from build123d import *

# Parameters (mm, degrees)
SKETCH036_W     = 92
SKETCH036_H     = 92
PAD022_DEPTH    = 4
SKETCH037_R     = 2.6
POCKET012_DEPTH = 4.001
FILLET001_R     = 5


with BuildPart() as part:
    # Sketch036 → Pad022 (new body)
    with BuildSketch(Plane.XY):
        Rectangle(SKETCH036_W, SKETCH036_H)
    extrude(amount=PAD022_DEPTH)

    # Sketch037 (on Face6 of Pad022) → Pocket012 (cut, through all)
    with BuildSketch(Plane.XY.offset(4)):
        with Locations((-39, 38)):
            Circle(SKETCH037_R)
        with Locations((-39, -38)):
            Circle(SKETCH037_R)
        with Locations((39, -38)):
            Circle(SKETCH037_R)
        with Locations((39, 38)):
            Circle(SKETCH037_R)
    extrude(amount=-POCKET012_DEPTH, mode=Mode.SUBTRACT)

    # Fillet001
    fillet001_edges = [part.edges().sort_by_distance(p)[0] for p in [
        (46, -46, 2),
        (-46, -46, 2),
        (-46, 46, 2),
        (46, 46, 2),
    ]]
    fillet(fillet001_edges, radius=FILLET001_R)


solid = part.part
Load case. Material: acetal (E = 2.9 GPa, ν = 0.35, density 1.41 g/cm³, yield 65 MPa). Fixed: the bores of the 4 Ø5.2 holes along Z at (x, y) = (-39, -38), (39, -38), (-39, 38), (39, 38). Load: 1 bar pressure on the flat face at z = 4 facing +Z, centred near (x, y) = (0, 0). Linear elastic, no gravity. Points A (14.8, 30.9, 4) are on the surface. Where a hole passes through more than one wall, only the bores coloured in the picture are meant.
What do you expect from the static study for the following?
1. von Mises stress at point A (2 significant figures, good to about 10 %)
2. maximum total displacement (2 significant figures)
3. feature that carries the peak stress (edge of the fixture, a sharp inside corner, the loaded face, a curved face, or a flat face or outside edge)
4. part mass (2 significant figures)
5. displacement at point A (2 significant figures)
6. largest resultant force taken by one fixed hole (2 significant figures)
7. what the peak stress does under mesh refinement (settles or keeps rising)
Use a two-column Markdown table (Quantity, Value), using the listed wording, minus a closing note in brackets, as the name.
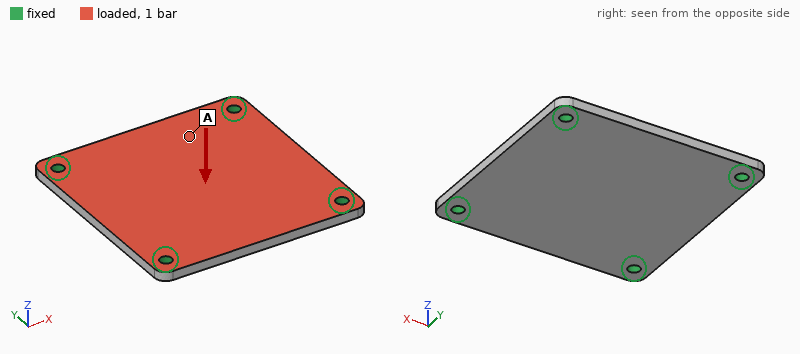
| Quantity | Value |
|---|---|
| von Mises stress at point A | 7.6 MPa |
| maximum total displacement | 1.5 mm |
| feature that carries the peak stress | edge of the fixture |
| part mass | 47 g |
| displacement at point A | 0.79 mm |
| largest resultant force taken by one fixed hole | 210 N |
| what the peak stress does under mesh refinement | keeps rising |
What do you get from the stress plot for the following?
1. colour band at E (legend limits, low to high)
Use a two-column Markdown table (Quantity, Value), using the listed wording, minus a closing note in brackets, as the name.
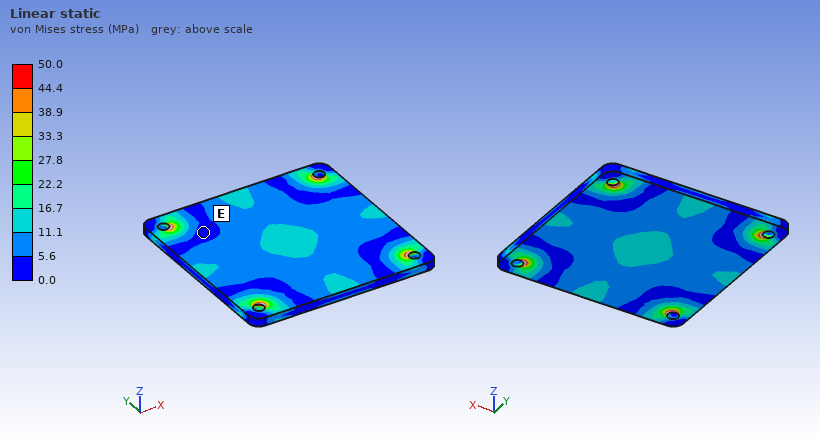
| Quantity | Value |
|---|---|
| colour band at E | 0.0 to 5.6 MPa |
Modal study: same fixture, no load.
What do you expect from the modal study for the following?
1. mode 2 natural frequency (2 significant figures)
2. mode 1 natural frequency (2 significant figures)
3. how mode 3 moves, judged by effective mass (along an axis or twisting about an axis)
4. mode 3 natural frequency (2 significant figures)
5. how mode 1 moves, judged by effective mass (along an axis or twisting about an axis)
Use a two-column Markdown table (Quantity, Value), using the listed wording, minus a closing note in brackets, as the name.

| Quantity | Value |
|---|---|
| mode 2 natural frequency | 1100 Hz |
| mode 1 natural frequency | 670 Hz |
| how mode 3 moves, judged by effective mass | twisting about Y |
| mode 3 natural frequency | 1100 Hz |
| how mode 1 moves, judged by effective mass | along Z |
